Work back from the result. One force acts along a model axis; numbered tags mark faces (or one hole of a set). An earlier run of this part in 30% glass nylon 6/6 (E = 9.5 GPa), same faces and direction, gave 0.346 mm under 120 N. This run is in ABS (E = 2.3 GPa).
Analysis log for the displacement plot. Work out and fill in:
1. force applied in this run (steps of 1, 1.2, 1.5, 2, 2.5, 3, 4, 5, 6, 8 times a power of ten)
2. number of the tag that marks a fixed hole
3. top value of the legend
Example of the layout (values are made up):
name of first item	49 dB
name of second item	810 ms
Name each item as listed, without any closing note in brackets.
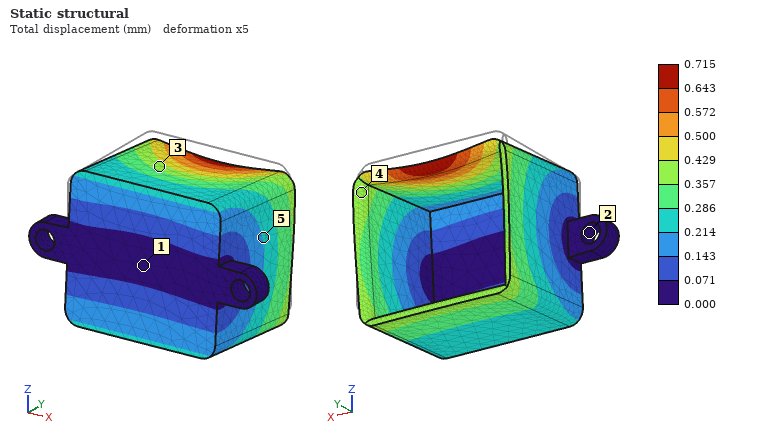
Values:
force applied in this run	60 N
number of the tag that marks a fixed hole	2
top value of the legend	0.715 mm
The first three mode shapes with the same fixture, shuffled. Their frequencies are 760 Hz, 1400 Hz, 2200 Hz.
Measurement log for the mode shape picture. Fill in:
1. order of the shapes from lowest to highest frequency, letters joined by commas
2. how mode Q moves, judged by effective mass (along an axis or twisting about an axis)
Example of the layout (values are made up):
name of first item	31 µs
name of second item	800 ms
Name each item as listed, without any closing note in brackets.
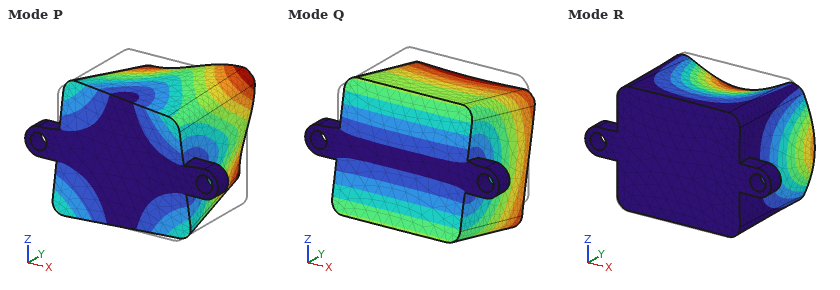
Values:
order of the shapes from lowest to highest frequency, letters joined by commas	Q, P, R
how mode Q moves, judged by effective mass	along Z
